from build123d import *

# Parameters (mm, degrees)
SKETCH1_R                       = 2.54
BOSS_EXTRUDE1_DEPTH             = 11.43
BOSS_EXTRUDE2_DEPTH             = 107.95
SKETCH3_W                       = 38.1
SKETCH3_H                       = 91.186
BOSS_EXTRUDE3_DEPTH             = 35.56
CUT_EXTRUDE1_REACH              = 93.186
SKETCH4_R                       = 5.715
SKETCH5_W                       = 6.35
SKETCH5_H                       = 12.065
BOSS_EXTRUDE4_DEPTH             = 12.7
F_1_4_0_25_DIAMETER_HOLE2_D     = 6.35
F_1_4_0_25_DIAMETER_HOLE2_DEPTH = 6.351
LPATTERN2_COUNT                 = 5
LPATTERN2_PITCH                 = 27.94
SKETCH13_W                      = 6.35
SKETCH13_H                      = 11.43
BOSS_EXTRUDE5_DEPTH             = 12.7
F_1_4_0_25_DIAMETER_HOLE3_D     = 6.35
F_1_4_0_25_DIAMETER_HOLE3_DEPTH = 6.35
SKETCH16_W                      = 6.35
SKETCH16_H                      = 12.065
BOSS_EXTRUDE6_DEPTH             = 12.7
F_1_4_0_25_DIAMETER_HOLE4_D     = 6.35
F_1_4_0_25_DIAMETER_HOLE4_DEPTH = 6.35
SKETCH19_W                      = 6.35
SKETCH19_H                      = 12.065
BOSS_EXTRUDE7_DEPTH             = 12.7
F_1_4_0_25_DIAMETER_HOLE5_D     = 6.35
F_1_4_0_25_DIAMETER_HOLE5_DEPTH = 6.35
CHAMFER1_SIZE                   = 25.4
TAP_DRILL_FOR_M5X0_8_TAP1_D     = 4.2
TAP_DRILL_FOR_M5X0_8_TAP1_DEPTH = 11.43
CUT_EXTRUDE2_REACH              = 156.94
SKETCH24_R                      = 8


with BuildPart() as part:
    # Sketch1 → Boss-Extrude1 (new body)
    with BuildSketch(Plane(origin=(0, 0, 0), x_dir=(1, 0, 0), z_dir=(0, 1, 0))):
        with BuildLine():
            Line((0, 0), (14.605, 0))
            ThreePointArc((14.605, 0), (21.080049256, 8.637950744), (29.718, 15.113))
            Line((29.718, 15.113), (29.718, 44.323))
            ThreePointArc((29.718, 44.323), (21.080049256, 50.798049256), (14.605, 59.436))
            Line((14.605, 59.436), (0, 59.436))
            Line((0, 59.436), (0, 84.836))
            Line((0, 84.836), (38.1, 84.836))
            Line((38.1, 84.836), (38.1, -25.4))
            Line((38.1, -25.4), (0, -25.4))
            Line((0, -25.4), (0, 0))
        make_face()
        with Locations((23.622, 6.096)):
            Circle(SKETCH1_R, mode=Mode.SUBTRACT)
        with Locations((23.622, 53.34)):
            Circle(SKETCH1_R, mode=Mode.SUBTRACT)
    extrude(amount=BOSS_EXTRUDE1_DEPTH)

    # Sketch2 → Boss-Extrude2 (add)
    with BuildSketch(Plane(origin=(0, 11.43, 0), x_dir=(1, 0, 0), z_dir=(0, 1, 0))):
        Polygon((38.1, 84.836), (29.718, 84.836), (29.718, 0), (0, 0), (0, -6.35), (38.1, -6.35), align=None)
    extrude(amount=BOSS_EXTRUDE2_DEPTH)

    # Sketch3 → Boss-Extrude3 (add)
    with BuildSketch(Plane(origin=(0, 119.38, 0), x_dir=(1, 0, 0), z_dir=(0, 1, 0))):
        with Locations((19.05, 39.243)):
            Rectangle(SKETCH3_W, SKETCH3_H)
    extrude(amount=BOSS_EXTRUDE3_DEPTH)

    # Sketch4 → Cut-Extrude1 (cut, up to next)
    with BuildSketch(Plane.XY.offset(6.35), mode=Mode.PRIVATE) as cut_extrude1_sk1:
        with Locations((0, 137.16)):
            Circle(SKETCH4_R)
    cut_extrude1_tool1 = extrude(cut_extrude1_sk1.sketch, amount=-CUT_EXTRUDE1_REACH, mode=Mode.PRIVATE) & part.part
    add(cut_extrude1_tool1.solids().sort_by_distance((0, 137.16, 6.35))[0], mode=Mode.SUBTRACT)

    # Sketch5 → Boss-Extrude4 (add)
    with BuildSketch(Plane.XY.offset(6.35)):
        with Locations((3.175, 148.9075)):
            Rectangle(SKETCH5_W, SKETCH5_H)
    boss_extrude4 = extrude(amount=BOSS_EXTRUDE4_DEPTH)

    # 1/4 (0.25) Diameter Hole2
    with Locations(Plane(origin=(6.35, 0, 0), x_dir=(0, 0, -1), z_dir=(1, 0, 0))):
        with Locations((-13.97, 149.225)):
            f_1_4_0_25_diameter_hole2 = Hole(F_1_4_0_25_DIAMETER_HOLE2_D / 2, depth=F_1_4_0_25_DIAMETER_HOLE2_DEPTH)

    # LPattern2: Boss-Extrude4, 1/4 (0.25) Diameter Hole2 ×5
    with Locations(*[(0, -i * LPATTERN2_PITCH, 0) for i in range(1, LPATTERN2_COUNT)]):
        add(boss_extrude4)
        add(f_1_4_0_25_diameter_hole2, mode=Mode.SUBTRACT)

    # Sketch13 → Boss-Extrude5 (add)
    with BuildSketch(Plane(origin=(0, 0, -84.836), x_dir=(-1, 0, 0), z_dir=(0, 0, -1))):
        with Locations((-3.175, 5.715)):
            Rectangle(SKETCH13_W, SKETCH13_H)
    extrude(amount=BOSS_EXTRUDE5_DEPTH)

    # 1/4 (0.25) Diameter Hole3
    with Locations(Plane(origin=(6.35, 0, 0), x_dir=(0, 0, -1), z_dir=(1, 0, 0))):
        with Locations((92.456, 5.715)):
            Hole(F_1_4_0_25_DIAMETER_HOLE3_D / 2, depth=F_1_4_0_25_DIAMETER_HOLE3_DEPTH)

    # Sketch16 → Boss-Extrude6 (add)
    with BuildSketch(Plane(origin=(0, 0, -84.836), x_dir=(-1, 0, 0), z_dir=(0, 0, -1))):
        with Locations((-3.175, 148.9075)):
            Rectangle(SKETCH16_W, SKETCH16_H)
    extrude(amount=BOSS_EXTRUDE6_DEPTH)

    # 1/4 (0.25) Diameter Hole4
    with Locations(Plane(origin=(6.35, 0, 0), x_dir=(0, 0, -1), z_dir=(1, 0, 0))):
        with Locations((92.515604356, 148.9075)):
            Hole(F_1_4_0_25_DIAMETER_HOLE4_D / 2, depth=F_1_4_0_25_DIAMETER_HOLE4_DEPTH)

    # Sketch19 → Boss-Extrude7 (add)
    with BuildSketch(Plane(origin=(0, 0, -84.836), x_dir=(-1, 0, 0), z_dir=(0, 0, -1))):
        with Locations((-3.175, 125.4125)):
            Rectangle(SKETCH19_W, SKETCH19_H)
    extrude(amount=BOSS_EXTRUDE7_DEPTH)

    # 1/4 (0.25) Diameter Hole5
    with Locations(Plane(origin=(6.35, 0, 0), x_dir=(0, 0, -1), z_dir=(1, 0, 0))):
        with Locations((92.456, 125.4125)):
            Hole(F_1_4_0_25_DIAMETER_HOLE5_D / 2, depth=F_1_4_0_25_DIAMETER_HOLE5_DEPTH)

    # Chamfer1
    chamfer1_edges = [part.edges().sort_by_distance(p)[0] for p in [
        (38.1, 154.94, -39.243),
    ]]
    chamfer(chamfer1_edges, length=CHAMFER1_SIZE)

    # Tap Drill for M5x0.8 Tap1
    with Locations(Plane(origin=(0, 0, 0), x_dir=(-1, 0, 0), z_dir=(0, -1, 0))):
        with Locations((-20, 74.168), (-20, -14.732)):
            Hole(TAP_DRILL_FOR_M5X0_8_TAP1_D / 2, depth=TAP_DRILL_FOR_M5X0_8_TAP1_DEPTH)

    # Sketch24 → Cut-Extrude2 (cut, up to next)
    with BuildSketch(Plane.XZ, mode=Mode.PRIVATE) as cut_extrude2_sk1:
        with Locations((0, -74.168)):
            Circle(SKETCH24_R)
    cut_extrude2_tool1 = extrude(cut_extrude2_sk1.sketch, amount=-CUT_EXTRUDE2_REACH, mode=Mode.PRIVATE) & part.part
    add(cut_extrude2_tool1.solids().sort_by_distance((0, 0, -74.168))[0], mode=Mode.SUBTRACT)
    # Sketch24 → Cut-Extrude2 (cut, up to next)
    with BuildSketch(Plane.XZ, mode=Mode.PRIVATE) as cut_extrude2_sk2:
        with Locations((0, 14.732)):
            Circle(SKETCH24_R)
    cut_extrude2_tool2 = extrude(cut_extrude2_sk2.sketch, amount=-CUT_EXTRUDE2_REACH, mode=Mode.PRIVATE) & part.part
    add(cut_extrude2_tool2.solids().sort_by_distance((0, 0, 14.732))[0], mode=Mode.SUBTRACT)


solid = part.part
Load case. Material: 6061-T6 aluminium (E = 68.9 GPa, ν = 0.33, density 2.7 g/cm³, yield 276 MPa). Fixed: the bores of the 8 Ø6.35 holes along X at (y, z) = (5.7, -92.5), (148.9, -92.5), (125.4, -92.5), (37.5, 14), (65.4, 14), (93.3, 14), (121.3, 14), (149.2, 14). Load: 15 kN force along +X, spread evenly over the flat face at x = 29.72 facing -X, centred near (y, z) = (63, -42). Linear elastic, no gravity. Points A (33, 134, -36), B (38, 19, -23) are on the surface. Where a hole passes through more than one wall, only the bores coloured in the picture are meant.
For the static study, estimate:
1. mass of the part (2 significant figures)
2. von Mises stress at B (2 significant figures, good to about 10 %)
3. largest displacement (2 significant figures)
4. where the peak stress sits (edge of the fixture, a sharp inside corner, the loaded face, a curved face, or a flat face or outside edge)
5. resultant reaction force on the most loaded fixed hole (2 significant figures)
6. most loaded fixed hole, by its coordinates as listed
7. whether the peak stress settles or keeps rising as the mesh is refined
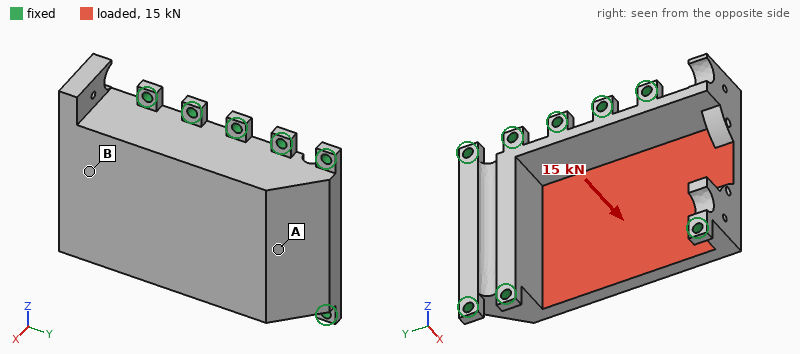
610 g
41 MPa
0.35 mm
edge of the fixture
5.1 kN
(5.7, -92.5)
keeps rising
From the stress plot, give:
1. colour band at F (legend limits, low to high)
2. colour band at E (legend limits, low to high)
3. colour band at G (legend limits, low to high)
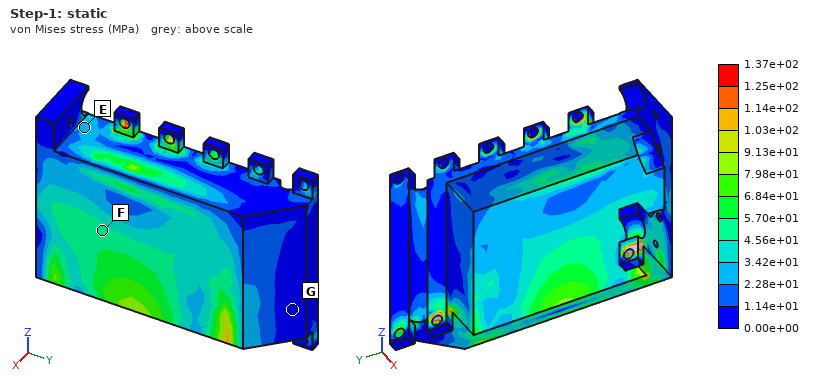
4.56e+01 to 5.70e+01 MPa
2.28e+01 to 3.42e+01 MPa
0.00e+00 to 1.14e+01 MPa
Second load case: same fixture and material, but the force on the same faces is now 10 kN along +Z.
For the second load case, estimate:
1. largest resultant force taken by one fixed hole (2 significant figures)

2.5 kN
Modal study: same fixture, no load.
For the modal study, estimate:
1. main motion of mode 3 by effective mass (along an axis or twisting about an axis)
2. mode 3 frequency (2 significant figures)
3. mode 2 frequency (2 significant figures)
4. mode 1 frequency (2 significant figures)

along Y
3500 Hz
3100 Hz
2700 Hz
